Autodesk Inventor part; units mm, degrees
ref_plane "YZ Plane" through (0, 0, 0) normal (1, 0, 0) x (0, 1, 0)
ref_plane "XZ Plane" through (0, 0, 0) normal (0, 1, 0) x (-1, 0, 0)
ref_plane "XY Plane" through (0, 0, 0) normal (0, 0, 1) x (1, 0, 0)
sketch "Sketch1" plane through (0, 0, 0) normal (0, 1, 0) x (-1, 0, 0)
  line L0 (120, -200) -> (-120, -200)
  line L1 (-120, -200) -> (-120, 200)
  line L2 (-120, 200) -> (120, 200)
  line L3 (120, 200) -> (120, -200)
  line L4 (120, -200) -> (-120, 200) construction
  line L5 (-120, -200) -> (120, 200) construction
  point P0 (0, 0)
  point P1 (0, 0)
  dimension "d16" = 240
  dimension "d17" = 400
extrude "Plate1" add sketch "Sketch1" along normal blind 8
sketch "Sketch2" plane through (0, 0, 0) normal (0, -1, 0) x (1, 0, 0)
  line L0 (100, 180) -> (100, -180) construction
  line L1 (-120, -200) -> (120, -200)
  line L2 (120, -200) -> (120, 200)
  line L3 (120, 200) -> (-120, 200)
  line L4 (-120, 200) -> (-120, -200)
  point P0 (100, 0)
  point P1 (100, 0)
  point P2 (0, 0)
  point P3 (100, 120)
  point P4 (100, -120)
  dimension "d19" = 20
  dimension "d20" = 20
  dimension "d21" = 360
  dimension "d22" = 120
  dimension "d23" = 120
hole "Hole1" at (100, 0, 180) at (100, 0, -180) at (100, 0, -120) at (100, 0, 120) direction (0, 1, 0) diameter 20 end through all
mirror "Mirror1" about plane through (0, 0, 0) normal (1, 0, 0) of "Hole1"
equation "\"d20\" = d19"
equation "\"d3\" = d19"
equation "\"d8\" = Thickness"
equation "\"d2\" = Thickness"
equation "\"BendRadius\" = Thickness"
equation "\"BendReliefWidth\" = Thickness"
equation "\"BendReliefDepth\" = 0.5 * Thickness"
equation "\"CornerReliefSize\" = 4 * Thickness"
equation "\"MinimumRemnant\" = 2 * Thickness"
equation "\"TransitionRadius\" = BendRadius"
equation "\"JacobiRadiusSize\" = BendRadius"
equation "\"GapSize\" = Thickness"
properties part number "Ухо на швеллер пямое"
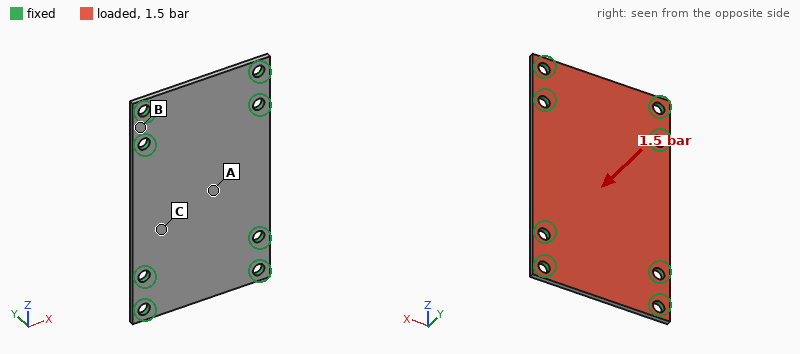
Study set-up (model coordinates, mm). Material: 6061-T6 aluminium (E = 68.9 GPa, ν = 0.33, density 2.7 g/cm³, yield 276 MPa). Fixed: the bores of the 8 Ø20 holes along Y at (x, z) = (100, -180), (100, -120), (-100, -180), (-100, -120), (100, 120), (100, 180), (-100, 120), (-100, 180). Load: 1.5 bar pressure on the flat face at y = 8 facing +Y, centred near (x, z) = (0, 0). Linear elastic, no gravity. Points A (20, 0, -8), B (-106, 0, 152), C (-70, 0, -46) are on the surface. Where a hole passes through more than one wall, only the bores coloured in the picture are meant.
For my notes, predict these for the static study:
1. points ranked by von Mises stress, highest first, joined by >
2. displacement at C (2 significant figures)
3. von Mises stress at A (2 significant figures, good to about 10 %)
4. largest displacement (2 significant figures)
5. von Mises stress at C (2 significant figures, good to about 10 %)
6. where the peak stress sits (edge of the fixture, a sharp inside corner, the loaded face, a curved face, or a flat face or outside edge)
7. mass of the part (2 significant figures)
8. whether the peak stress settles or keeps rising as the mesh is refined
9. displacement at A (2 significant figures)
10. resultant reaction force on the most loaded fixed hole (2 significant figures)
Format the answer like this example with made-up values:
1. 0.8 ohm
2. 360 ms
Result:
1. A > C > B
2. 0.42 mm
3. 32 MPa
4. 0.66 mm
5. 21 MPa
6. edge of the fixture
7. 2.0 kg
8. keeps rising
9. 0.65 mm
10. 2.9 kN
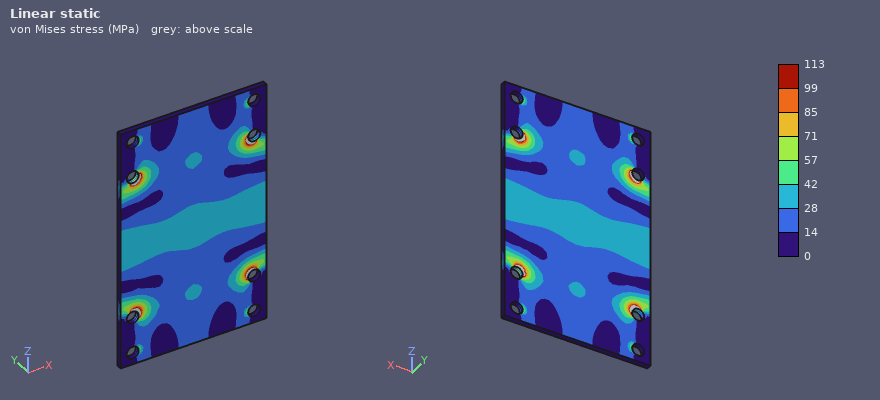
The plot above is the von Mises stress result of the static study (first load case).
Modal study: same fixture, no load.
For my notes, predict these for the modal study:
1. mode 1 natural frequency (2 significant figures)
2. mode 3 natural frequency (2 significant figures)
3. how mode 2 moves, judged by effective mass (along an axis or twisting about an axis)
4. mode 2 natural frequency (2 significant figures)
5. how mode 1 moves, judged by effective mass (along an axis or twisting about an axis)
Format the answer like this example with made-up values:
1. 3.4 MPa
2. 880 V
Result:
1. 630 Hz
2. 1200 Hz
3. twisting about Z
4. 940 Hz
5. along Y
